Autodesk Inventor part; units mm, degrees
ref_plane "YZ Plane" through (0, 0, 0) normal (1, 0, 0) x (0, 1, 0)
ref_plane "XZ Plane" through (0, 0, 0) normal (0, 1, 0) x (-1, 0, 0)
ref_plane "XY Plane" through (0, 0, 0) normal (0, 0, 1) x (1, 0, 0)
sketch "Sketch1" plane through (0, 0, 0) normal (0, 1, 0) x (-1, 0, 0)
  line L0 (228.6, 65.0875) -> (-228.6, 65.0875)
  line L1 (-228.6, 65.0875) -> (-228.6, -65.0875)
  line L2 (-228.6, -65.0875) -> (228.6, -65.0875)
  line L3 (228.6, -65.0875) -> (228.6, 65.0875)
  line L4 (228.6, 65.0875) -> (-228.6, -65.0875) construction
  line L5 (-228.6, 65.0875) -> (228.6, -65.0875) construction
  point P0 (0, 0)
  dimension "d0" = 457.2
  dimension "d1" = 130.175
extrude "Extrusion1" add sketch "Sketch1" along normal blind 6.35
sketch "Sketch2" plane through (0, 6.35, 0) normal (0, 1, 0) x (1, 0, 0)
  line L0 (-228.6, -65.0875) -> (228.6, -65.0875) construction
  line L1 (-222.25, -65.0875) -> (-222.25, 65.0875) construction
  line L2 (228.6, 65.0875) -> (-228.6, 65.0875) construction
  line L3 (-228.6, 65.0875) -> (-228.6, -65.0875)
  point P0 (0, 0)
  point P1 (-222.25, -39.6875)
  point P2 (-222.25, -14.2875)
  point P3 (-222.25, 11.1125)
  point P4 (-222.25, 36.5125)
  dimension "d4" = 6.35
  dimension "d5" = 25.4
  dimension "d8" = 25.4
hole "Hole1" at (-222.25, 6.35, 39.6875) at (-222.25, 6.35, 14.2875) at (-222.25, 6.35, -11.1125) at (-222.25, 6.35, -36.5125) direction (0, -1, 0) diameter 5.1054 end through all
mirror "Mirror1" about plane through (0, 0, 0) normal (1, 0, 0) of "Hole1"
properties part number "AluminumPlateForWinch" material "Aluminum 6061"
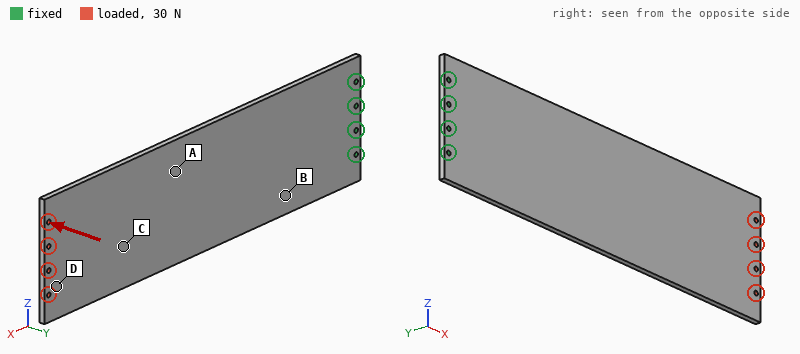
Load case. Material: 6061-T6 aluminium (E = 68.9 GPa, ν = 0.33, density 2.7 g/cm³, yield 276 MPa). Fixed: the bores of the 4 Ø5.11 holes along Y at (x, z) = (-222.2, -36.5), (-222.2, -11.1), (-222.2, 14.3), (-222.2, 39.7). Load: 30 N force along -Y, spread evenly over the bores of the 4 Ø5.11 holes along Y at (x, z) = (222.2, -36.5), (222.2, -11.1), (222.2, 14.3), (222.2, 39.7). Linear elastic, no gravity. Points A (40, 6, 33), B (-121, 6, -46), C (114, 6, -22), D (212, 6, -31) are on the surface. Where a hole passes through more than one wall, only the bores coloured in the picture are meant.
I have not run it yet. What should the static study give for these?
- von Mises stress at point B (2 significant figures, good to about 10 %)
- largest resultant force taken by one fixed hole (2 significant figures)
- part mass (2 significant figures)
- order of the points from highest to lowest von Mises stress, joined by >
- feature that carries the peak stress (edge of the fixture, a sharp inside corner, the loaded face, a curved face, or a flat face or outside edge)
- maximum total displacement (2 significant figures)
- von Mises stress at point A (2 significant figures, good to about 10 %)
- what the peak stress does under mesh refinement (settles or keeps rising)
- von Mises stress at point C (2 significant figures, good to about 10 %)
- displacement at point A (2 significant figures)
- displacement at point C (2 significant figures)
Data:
12 MPa
49 N
1.0 kg
B > A > C > D
edge of the fixture
4.7 mm
6.3 MPa
keeps rising
3.8 MPa
1.9 mm
2.9 mm
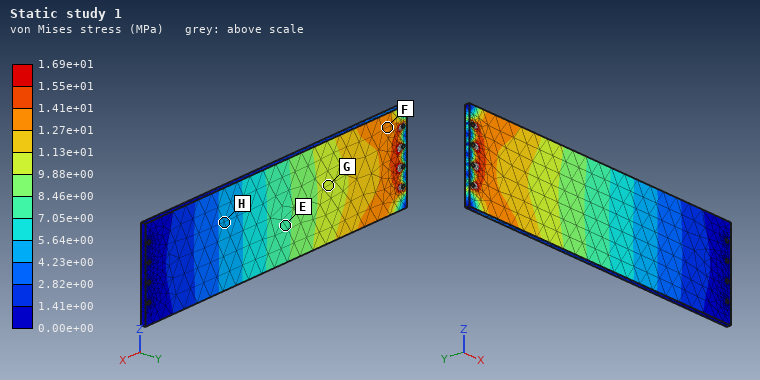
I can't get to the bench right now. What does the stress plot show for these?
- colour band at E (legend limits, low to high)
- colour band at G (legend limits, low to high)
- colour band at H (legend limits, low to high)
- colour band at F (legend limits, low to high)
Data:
7.05e+00 to 8.46e+00 MPa
9.88e+00 to 1.13e+01 MPa
4.23e+00 to 5.64e+00 MPa
1.27e+01 to 1.41e+01 MPa
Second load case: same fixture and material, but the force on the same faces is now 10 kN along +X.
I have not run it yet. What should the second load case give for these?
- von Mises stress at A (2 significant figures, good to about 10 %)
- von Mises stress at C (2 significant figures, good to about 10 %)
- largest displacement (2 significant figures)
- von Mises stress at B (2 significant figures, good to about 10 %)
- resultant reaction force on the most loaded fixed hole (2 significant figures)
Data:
13 MPa
12 MPa
91 µm
11 MPa
2.9 kN
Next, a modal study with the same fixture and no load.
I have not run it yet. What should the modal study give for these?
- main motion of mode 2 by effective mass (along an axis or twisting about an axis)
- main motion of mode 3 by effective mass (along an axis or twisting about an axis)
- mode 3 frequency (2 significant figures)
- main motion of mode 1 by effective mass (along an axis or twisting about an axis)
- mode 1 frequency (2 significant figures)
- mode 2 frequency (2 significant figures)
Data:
along Y
twisting about X
180 Hz
along Y
26 Hz
160 Hz
